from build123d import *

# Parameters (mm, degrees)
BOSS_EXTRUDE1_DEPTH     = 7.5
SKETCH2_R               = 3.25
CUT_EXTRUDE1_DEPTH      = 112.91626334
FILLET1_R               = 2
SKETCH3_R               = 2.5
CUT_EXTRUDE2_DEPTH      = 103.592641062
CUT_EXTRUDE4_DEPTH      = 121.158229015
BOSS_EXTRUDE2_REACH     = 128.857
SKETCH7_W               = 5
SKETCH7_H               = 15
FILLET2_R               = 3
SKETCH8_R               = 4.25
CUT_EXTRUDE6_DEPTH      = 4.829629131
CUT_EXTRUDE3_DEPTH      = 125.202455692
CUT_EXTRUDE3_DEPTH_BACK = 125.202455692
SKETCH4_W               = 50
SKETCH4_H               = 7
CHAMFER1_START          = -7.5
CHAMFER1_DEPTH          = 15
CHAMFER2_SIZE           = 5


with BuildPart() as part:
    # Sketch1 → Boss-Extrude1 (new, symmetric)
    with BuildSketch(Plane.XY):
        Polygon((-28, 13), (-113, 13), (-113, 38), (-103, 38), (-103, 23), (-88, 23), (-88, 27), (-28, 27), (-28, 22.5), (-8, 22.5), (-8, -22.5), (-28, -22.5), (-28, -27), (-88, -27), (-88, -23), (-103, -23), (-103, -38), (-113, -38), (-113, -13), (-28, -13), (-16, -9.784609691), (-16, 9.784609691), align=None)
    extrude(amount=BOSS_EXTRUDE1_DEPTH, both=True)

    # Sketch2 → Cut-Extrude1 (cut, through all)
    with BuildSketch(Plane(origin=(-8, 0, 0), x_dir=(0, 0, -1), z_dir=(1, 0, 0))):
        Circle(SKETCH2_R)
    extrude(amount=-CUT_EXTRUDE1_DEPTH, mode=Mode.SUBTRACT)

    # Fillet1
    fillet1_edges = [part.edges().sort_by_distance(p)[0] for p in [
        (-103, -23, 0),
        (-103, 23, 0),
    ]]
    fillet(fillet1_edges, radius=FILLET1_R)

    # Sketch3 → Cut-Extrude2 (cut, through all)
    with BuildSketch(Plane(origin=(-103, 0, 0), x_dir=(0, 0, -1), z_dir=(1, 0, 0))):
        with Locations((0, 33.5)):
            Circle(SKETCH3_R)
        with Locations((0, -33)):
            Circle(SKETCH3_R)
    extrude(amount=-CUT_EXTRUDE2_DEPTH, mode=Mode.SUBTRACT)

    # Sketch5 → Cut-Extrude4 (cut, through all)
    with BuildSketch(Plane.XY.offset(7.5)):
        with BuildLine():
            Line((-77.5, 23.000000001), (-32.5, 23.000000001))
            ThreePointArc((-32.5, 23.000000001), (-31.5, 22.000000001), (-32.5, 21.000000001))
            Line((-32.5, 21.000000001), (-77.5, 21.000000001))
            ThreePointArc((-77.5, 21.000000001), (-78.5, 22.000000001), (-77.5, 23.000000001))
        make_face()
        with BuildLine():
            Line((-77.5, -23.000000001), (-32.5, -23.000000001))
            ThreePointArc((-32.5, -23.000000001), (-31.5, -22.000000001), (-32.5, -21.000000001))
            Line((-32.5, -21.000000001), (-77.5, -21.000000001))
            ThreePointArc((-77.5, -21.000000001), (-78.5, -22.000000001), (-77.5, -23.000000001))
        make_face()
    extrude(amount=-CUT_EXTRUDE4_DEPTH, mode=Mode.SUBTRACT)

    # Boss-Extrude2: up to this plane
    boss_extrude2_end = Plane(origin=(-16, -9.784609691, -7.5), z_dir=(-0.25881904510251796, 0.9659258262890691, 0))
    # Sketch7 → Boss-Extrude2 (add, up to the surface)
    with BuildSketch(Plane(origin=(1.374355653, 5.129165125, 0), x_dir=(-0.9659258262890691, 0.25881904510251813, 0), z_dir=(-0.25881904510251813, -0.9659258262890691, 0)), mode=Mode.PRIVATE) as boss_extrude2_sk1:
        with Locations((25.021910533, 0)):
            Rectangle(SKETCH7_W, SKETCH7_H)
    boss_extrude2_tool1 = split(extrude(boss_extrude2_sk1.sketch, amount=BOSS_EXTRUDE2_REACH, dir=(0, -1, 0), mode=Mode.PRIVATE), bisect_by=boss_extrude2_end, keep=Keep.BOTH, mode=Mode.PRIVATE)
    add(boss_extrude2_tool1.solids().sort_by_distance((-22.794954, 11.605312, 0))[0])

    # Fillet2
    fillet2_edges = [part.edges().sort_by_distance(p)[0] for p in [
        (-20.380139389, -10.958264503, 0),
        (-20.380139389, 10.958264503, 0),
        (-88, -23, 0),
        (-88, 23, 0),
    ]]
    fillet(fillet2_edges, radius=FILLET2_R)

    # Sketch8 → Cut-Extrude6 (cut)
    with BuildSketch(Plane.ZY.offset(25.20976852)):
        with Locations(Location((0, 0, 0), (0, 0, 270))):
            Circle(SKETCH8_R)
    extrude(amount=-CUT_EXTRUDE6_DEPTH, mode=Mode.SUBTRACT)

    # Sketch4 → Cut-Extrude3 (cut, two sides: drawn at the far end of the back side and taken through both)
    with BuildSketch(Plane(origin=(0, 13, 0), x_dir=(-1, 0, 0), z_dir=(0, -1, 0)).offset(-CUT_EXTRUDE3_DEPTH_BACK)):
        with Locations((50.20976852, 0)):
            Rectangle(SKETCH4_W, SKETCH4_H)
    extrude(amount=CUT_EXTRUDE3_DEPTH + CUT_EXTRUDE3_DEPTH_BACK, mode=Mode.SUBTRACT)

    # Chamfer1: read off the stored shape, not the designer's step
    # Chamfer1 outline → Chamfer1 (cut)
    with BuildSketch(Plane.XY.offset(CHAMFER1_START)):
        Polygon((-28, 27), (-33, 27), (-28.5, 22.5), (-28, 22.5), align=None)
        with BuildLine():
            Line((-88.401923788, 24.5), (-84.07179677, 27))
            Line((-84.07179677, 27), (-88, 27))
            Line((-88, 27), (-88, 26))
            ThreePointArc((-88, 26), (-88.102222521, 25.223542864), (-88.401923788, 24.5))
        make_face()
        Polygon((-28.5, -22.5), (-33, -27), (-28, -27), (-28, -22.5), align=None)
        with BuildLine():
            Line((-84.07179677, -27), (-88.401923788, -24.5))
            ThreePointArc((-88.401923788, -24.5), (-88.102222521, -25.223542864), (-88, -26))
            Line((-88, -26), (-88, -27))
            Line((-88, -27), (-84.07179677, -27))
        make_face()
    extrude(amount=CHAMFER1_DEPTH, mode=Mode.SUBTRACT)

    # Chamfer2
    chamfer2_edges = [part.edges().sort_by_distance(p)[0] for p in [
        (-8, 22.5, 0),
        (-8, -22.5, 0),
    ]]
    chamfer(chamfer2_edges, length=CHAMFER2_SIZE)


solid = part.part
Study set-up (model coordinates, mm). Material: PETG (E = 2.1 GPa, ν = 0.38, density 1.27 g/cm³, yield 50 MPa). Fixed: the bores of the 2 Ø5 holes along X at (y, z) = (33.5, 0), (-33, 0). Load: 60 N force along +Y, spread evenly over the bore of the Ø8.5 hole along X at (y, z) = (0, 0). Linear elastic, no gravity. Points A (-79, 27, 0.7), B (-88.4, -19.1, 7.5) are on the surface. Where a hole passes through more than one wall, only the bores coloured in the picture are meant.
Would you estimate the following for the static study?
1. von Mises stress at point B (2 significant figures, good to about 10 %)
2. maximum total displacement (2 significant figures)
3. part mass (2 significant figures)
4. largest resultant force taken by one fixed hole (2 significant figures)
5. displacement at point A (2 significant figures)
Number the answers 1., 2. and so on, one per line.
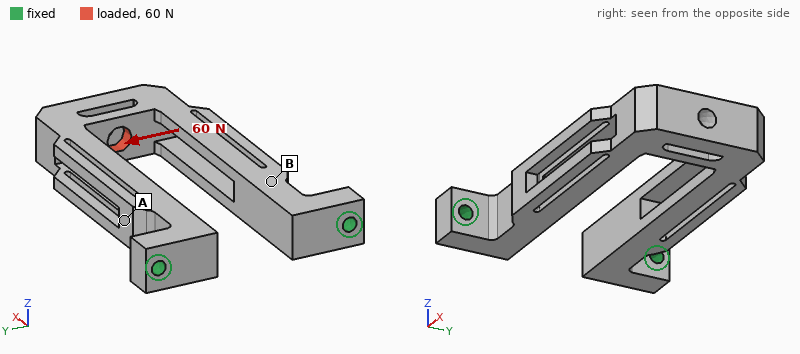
1. 1.7 MPa
2. 1.2 mm
3. 45 g
4. 69 N
5. 0.28 mm
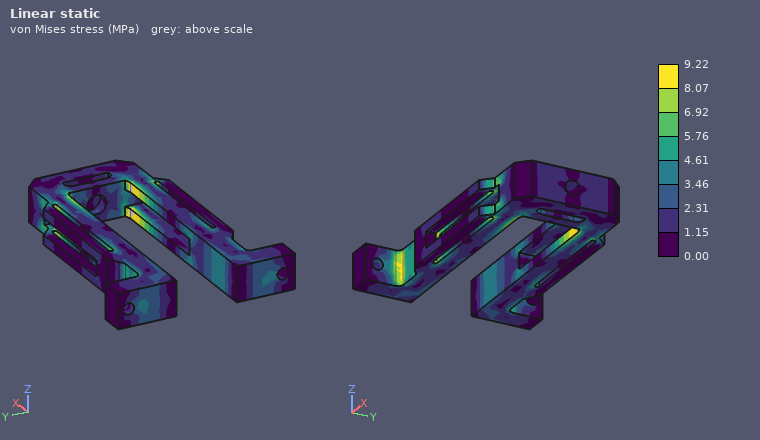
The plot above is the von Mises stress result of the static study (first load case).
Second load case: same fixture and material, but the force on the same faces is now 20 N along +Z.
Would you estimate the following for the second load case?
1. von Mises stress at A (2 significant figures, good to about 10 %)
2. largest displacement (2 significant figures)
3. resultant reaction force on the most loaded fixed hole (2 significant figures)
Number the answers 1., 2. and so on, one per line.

1. 0.58 MPa
2. 1.3 mm
3. 10 N
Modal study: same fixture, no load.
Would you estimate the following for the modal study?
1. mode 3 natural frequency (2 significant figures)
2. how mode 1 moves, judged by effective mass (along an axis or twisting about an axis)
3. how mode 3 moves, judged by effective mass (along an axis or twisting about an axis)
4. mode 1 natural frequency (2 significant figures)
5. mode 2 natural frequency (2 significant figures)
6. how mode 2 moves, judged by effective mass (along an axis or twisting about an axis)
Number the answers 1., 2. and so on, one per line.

1. 350 Hz
2. along Z
3. twisting about X
4. 150 Hz
5. 260 Hz
6. along Y
